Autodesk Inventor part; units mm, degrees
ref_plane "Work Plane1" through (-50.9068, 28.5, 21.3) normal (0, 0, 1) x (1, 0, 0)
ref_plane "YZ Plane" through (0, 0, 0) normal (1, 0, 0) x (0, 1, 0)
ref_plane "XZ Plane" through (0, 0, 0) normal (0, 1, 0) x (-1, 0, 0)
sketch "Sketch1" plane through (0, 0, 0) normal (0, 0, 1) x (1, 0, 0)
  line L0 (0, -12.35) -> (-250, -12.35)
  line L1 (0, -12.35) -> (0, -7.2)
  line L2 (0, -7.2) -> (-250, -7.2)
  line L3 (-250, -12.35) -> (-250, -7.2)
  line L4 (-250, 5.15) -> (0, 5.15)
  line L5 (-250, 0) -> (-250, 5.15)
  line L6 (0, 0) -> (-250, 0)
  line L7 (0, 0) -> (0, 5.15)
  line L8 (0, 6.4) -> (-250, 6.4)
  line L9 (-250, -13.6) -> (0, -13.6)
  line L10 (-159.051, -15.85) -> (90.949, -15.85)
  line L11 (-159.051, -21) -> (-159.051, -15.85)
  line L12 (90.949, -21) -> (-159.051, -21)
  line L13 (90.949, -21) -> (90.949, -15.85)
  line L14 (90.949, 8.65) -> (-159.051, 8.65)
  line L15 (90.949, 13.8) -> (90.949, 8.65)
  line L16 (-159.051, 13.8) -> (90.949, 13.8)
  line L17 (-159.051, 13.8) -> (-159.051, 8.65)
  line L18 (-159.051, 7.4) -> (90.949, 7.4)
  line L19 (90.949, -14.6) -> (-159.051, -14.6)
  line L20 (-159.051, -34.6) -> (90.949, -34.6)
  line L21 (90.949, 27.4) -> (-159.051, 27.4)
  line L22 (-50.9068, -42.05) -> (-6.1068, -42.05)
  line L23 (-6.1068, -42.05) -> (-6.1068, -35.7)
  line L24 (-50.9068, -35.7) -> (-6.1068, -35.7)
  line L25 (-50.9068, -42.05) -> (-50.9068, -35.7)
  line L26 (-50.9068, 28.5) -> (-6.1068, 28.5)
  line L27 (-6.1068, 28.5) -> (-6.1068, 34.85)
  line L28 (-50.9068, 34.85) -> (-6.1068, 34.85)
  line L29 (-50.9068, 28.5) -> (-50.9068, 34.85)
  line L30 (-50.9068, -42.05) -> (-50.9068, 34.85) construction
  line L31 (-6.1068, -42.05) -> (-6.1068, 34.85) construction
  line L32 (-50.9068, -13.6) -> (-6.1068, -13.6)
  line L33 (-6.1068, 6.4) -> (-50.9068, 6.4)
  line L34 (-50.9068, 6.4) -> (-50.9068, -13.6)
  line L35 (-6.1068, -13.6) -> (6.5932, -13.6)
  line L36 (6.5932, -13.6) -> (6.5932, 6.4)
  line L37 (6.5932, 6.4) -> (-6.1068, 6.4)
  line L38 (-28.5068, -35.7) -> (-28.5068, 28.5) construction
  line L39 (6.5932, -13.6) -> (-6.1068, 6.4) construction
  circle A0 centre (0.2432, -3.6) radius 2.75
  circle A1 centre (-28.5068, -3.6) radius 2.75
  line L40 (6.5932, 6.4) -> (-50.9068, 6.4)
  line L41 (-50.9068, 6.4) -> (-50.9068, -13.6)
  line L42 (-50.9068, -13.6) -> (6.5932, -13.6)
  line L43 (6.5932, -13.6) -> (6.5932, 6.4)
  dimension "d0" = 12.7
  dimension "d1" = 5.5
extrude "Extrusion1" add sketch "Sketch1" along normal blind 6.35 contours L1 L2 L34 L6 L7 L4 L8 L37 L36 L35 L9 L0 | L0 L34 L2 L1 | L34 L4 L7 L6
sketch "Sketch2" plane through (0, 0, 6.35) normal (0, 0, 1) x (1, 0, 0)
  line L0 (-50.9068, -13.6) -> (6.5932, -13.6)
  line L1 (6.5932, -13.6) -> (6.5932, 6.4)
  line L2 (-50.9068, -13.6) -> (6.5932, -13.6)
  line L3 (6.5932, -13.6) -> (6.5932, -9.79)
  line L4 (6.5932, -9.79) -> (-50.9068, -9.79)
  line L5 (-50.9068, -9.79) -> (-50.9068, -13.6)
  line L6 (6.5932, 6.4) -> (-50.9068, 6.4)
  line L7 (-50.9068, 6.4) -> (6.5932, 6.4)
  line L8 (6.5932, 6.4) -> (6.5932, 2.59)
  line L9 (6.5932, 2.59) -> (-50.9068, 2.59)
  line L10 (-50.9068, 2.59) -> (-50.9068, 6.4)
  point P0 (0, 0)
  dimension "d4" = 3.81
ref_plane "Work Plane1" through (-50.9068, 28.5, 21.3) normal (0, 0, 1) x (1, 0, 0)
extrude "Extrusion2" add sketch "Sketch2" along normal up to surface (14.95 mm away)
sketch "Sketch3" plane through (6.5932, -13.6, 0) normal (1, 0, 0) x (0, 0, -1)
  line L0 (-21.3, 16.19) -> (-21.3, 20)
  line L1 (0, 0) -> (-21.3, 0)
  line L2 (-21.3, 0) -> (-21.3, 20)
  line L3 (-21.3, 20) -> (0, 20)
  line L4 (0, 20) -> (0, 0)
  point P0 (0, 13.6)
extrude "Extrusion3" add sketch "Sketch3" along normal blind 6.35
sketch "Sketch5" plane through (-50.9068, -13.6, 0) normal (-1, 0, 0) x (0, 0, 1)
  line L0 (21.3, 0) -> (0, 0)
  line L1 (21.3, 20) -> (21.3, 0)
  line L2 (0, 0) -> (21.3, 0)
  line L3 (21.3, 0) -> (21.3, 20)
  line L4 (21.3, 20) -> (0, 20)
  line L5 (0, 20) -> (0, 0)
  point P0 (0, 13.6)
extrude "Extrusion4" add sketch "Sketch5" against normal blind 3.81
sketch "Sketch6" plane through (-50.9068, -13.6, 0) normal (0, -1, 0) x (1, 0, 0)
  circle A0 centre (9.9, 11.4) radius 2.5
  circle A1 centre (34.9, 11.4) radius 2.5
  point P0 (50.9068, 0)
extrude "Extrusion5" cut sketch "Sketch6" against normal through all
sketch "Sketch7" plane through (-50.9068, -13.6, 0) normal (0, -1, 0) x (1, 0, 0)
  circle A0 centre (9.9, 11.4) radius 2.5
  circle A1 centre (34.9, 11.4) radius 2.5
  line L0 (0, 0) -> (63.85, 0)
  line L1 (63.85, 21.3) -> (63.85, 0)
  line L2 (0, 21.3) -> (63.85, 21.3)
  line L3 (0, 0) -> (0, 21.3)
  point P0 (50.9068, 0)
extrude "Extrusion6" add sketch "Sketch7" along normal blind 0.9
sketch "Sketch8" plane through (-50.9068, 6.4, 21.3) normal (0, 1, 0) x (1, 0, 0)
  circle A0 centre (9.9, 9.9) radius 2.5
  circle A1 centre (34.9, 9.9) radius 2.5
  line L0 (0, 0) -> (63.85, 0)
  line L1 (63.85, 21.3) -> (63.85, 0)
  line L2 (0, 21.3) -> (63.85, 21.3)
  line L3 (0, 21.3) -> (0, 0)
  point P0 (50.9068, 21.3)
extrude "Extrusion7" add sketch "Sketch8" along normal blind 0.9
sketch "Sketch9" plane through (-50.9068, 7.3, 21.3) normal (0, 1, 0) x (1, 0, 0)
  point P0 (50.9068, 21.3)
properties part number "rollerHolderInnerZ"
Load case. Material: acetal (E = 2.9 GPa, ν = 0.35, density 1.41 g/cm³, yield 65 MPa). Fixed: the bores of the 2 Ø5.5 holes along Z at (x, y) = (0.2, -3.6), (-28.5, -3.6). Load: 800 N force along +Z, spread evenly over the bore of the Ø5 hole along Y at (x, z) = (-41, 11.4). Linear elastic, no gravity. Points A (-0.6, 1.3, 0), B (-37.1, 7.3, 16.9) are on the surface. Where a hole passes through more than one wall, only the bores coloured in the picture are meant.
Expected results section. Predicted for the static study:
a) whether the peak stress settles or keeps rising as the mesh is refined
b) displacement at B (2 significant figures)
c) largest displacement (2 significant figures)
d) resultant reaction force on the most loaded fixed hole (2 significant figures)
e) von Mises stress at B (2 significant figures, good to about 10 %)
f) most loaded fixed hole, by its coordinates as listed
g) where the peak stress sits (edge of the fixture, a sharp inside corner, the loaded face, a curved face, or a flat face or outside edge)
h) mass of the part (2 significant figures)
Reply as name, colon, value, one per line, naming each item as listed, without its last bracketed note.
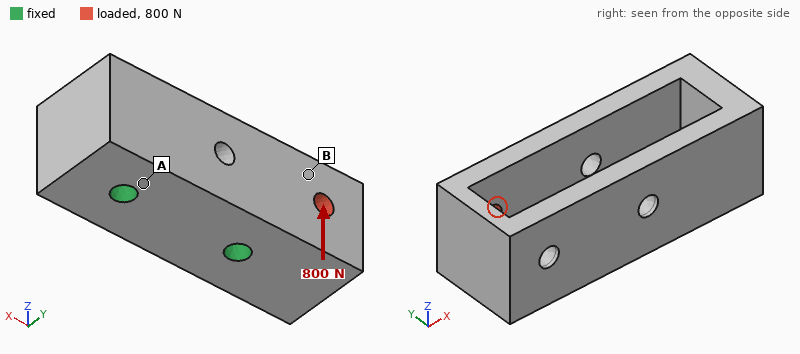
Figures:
whether the peak stress settles or keeps rising as the mesh is refined: keeps rising
displacement at B: 0.46 mm
largest displacement: 0.67 mm
resultant reaction force on the most loaded fixed hole: 1.0 kN
von Mises stress at B: 14 MPa
most loaded fixed hole, by its coordinates as listed: (-28.5, -3.6)
where the peak stress sits: edge of the fixture
mass of the part: 27 g
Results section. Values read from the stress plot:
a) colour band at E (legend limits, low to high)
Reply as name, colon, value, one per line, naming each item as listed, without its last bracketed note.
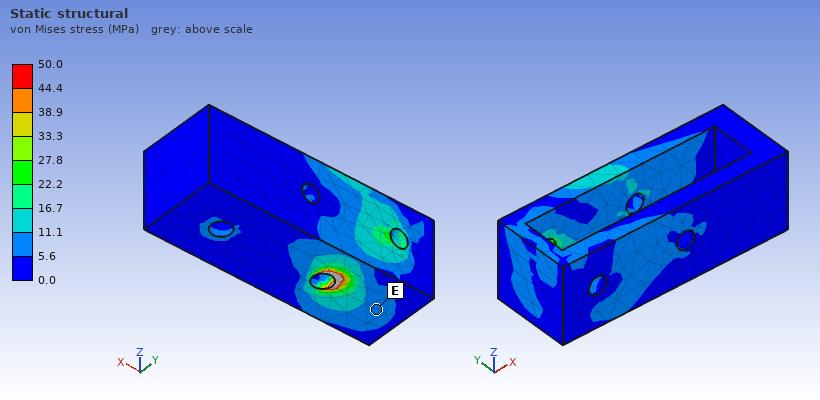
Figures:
colour band at E: 5.6 to 11.1 MPa
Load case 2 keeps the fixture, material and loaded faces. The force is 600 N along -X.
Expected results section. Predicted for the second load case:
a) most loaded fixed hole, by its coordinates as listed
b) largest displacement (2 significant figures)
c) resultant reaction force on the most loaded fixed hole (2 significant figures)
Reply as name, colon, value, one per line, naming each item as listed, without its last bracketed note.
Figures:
most loaded fixed hole, by its coordinates as listed: (-28.5, -3.6)
largest displacement: 0.14 mm
resultant reaction force on the most loaded fixed hole: 430 N
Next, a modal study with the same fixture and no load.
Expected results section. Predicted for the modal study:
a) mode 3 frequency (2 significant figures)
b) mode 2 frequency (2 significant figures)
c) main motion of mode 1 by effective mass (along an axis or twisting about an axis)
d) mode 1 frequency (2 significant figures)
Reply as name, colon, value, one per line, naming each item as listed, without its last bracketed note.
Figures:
mode 3 frequency: 3100 Hz
mode 2 frequency: 2900 Hz
main motion of mode 1 by effective mass: along Y
mode 1 frequency: 2200 Hz
